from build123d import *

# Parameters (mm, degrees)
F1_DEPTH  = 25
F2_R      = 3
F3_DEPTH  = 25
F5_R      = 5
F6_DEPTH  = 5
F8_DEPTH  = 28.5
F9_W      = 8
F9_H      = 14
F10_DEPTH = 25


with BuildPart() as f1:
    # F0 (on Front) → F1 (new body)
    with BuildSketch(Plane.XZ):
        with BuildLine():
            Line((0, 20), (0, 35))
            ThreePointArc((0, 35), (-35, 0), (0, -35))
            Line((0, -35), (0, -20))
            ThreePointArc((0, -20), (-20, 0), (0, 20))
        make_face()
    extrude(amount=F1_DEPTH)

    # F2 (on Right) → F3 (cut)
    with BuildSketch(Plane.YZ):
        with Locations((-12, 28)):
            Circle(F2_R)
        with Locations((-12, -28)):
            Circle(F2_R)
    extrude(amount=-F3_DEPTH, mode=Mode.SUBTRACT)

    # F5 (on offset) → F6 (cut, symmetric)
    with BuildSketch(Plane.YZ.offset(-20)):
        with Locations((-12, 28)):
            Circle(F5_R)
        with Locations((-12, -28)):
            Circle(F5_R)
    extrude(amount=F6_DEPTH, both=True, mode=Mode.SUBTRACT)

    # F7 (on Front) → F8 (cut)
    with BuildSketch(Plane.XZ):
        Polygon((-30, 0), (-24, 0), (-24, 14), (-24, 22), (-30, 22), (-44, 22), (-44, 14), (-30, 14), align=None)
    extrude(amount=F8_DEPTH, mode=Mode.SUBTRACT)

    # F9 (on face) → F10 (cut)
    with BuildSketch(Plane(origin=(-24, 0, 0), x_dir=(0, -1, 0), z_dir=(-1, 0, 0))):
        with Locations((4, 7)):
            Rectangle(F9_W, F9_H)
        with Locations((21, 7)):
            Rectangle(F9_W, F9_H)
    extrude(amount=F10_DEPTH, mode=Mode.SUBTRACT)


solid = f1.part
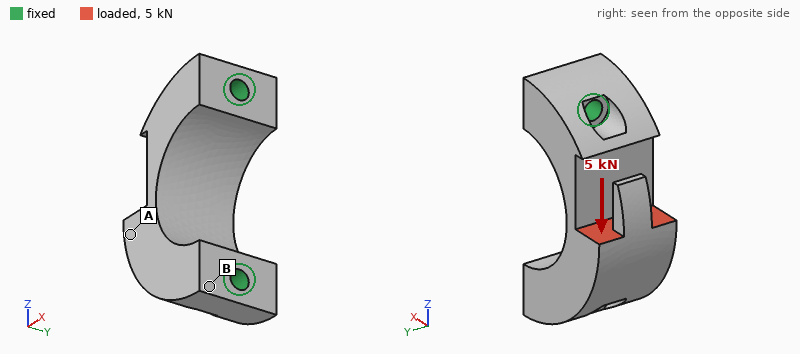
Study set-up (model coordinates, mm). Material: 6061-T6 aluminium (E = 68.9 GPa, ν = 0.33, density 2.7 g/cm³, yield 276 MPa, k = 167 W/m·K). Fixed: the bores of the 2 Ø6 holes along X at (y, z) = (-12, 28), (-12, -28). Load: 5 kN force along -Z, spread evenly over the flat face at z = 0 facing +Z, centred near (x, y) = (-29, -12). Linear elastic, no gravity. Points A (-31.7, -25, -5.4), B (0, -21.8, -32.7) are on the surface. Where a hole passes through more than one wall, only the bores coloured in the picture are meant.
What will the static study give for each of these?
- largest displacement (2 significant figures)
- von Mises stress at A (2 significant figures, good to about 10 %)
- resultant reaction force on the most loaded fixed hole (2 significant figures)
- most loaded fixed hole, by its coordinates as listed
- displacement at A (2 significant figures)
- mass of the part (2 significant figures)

33 µm
21 MPa
3.4 kN
(-12, 28)
22 µm
72 g
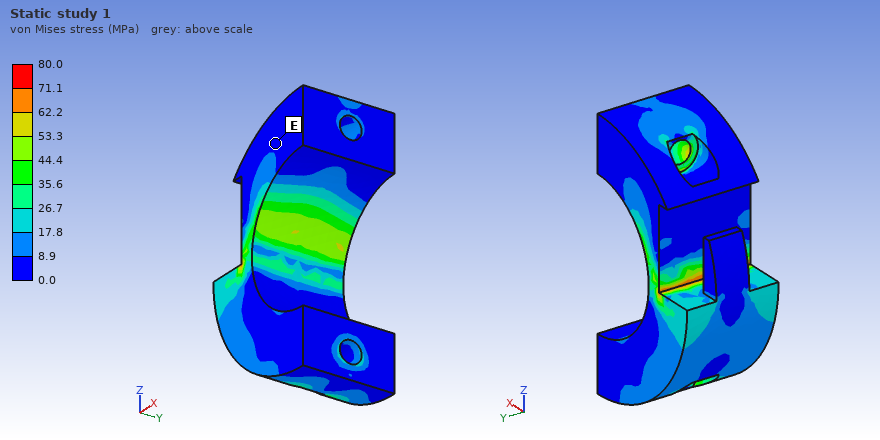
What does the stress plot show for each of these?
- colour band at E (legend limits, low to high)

0.0 to 8.9 MPa
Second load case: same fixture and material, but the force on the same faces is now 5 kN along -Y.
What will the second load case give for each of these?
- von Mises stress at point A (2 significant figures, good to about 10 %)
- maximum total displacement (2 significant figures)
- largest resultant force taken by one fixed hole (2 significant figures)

29 MPa
88 µm
2.6 kN
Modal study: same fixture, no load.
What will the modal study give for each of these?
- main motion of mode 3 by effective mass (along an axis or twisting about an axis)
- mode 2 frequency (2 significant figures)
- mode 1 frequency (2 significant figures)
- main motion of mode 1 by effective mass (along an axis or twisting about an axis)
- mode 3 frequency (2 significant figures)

along Z
13 kHz
10000 Hz
along Y
19 kHz
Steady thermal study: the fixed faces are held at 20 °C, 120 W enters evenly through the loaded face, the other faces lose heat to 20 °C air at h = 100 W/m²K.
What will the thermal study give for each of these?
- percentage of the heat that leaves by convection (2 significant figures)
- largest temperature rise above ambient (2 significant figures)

10 %
58 K
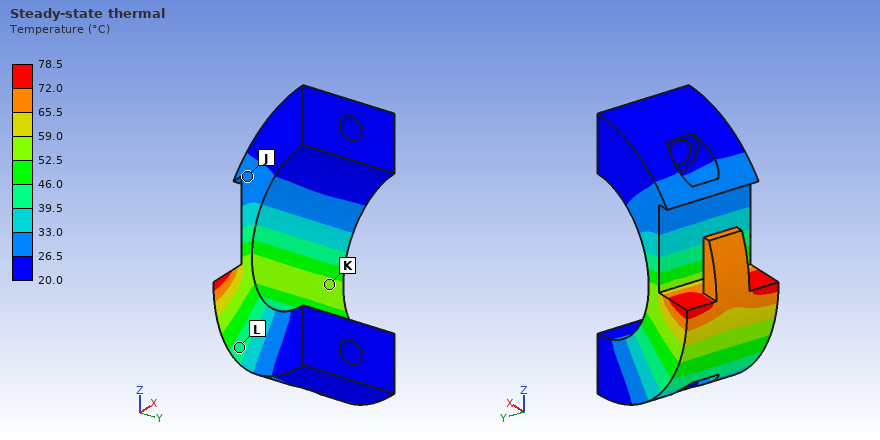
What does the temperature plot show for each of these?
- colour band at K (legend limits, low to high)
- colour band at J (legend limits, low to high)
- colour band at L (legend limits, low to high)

52.5 to 59.0 °C
26.5 to 33.0 °C
39.5 to 46.0 °C
